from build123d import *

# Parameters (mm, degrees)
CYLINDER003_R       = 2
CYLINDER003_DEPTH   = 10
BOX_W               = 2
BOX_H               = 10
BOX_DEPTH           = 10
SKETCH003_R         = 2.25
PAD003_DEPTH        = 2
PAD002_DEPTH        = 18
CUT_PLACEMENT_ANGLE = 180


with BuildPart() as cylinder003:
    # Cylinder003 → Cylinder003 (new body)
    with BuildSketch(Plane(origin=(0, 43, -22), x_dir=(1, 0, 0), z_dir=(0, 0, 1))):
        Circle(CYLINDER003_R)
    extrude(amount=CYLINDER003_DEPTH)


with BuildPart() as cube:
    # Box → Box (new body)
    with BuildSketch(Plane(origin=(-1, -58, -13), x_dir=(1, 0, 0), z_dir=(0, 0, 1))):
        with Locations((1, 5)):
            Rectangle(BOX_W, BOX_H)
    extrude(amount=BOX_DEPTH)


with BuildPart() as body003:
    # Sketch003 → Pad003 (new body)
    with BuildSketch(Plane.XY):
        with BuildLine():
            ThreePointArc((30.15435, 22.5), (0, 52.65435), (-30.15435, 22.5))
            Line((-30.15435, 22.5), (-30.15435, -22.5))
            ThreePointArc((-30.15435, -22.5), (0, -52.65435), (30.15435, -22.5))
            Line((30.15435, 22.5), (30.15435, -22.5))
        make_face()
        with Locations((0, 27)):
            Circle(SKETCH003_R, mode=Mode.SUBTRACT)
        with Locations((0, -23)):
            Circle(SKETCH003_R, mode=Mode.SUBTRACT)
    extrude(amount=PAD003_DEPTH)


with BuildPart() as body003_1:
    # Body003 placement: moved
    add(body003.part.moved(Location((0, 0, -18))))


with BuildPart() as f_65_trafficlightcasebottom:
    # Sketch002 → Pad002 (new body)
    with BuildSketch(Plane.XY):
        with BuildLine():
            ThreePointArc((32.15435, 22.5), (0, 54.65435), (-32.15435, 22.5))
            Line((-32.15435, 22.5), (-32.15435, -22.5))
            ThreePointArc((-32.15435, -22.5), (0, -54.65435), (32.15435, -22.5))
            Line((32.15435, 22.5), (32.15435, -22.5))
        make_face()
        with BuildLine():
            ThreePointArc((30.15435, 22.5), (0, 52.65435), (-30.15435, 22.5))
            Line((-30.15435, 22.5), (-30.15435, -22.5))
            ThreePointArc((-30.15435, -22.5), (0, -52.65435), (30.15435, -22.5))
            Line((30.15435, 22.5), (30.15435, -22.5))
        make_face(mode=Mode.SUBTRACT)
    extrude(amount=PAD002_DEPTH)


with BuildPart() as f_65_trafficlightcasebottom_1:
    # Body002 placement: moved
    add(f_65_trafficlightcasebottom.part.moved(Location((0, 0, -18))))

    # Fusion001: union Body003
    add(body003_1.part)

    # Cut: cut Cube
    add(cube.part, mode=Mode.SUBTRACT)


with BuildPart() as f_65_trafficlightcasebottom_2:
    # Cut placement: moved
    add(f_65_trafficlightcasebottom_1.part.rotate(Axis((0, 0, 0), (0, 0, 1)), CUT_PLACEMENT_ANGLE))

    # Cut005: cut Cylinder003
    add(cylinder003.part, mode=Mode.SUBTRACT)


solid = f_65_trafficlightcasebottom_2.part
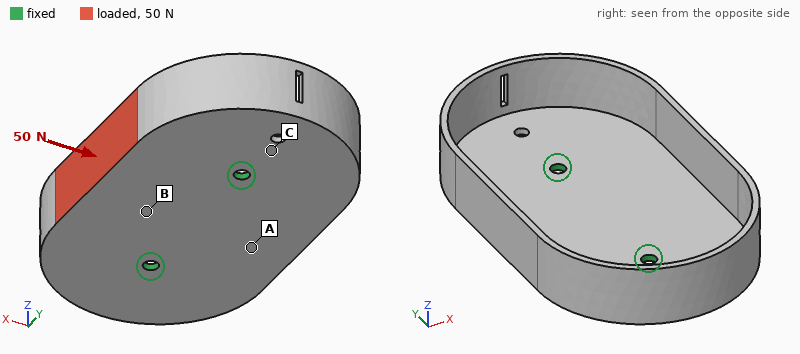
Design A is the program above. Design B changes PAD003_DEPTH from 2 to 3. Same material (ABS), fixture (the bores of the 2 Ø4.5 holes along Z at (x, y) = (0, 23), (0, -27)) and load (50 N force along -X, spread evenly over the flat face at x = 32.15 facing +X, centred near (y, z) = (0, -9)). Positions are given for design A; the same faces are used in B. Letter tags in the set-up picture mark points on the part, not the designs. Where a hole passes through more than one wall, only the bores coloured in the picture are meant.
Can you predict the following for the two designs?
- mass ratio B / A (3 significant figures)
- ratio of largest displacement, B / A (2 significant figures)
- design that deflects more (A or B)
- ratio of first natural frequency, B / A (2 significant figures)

1.26
0.43
A
1.6
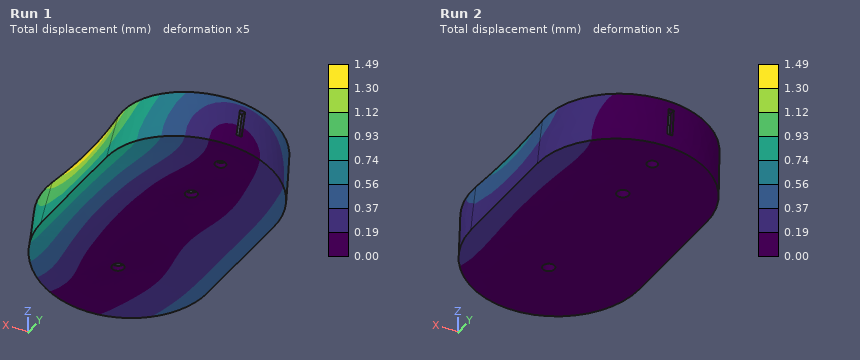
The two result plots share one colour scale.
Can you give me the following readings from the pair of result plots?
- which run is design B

Run 2
